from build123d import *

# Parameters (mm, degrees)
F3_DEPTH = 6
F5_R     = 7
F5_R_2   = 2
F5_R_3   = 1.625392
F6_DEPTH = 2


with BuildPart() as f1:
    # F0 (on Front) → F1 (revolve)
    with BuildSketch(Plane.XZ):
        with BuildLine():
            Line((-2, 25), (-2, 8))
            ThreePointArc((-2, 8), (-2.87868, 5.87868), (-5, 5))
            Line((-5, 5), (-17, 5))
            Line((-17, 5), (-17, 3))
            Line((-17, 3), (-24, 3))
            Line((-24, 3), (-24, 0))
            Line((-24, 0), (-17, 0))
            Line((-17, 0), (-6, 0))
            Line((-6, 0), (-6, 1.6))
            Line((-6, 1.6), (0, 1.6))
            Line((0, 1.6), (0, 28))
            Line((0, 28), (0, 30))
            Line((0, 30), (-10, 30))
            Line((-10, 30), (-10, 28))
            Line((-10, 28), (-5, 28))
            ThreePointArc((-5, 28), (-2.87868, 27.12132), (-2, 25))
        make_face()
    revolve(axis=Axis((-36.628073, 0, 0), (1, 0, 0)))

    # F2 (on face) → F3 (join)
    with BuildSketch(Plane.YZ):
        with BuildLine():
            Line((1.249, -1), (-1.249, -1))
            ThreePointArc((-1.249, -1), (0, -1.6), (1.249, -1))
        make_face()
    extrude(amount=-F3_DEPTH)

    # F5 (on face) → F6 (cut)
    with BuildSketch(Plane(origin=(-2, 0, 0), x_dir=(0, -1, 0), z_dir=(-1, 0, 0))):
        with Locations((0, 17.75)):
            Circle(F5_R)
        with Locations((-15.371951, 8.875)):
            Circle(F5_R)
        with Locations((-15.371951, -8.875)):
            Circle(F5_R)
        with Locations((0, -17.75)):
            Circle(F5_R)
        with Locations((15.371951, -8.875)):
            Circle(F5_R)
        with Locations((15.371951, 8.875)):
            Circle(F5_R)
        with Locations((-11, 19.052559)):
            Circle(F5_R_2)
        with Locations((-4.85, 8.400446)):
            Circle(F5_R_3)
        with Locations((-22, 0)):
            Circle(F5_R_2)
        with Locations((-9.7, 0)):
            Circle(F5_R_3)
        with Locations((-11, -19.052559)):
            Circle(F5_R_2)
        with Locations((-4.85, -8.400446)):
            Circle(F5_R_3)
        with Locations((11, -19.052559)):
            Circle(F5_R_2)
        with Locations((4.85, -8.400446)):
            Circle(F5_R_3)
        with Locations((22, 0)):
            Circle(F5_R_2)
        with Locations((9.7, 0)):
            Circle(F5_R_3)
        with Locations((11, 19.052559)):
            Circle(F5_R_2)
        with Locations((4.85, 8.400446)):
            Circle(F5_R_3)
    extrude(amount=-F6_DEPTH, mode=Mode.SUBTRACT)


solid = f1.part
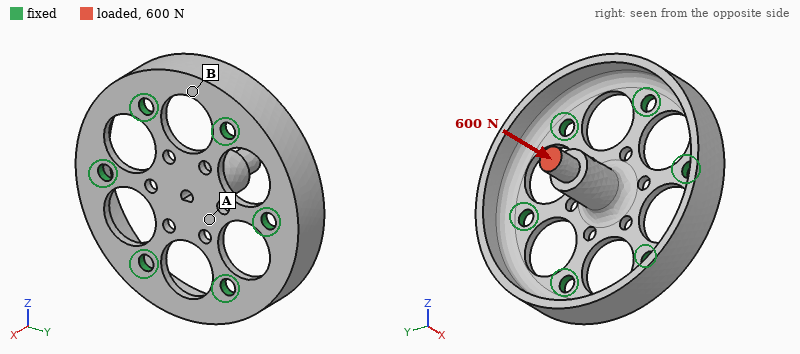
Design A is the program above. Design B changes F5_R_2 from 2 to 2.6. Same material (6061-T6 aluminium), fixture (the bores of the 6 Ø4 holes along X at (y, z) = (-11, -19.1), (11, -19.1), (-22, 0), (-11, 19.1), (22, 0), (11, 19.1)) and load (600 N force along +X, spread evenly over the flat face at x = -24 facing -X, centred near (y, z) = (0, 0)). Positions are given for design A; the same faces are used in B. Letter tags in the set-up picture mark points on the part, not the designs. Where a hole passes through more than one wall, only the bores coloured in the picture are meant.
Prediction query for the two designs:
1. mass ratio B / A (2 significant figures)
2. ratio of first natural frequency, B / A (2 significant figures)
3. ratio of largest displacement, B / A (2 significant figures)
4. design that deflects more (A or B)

0.99
1.0
0.90
A
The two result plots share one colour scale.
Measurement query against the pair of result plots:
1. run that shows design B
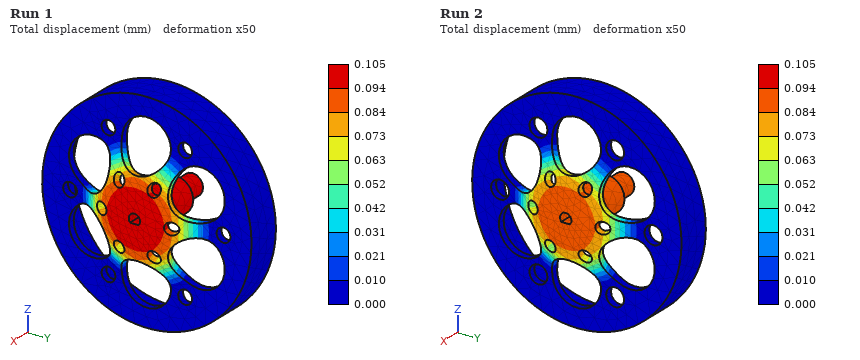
Run 2
